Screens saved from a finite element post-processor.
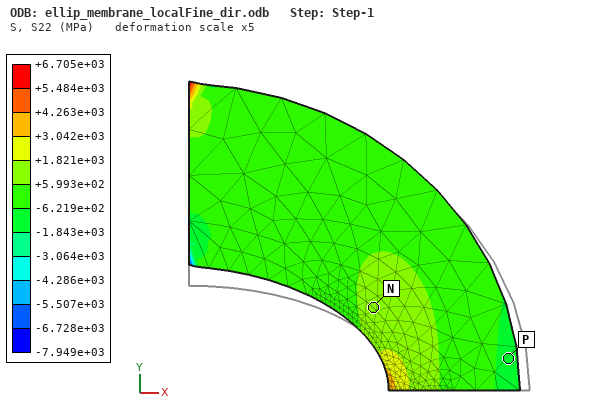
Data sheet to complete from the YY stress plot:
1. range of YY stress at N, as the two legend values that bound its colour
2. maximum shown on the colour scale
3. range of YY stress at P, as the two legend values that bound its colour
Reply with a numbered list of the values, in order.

1. +5.993e+02 to +1.821e+03 MPa
2. +6.705e+03 MPa
3. -1.843e+03 to -6.219e+02 MPa
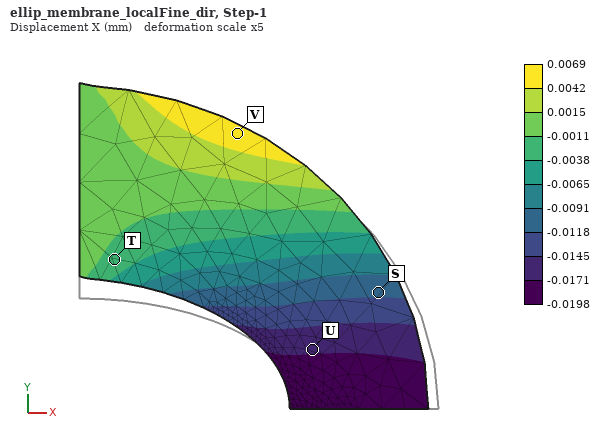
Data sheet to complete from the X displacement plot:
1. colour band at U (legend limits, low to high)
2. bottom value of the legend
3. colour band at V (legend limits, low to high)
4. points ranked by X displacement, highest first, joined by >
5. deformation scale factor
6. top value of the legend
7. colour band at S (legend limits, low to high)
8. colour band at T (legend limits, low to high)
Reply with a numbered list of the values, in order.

1. -0.0171 to -0.0145 mm
2. -0.0198 mm
3. 0.0042 to 0.0069 mm
4. V > T > S > U
5. 5
6. 0.0069 mm
7. -0.0118 to -0.0091 mm
8. -0.0038 to -0.0011 mm
